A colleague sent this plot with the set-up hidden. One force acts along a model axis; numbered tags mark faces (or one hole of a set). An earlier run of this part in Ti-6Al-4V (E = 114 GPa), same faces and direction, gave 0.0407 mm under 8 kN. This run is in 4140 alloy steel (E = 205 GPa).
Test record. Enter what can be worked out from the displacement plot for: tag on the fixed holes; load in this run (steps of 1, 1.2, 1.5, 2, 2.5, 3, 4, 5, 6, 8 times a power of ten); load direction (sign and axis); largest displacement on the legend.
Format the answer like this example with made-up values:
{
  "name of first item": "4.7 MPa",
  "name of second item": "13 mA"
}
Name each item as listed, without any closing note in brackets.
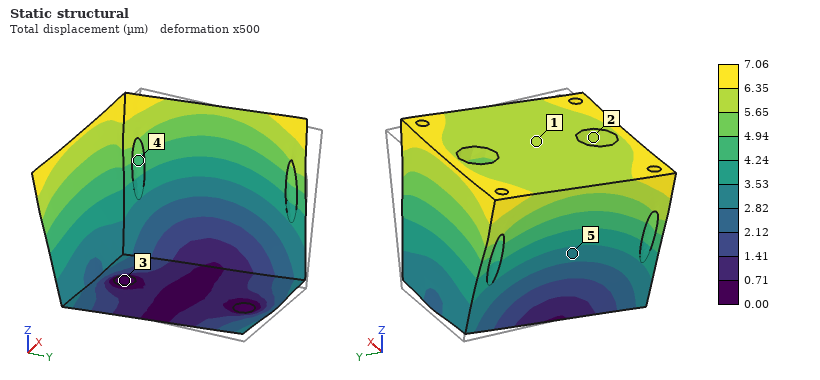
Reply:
{
  "tag on the fixed holes": "3",
  "load in this run": "2.5 kN",
  "load direction": "-Y",
  "largest displacement on the legend": "7.06 µm"
}
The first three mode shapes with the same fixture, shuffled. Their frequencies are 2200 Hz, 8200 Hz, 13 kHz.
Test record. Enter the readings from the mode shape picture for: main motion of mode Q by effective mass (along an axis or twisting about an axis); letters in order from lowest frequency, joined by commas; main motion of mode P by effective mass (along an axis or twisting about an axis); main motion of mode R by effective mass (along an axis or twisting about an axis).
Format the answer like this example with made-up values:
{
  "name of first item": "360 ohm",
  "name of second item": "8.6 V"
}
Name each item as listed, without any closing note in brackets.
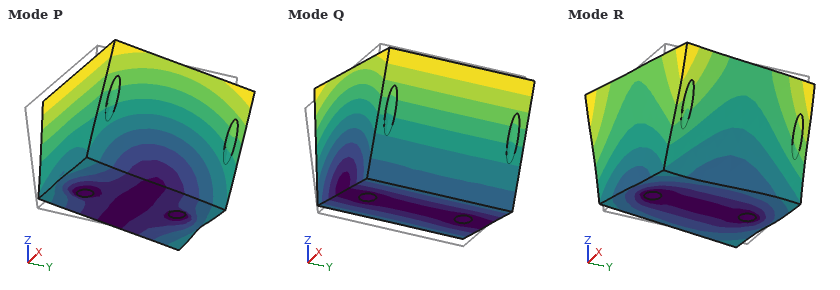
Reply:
{
  "main motion of mode Q by effective mass": "along X",
  "letters in order from lowest frequency, joined by commas": "Q, P, R",
  "main motion of mode P by effective mass": "along Y",
  "main motion of mode R by effective mass": "twisting about Z"
}
